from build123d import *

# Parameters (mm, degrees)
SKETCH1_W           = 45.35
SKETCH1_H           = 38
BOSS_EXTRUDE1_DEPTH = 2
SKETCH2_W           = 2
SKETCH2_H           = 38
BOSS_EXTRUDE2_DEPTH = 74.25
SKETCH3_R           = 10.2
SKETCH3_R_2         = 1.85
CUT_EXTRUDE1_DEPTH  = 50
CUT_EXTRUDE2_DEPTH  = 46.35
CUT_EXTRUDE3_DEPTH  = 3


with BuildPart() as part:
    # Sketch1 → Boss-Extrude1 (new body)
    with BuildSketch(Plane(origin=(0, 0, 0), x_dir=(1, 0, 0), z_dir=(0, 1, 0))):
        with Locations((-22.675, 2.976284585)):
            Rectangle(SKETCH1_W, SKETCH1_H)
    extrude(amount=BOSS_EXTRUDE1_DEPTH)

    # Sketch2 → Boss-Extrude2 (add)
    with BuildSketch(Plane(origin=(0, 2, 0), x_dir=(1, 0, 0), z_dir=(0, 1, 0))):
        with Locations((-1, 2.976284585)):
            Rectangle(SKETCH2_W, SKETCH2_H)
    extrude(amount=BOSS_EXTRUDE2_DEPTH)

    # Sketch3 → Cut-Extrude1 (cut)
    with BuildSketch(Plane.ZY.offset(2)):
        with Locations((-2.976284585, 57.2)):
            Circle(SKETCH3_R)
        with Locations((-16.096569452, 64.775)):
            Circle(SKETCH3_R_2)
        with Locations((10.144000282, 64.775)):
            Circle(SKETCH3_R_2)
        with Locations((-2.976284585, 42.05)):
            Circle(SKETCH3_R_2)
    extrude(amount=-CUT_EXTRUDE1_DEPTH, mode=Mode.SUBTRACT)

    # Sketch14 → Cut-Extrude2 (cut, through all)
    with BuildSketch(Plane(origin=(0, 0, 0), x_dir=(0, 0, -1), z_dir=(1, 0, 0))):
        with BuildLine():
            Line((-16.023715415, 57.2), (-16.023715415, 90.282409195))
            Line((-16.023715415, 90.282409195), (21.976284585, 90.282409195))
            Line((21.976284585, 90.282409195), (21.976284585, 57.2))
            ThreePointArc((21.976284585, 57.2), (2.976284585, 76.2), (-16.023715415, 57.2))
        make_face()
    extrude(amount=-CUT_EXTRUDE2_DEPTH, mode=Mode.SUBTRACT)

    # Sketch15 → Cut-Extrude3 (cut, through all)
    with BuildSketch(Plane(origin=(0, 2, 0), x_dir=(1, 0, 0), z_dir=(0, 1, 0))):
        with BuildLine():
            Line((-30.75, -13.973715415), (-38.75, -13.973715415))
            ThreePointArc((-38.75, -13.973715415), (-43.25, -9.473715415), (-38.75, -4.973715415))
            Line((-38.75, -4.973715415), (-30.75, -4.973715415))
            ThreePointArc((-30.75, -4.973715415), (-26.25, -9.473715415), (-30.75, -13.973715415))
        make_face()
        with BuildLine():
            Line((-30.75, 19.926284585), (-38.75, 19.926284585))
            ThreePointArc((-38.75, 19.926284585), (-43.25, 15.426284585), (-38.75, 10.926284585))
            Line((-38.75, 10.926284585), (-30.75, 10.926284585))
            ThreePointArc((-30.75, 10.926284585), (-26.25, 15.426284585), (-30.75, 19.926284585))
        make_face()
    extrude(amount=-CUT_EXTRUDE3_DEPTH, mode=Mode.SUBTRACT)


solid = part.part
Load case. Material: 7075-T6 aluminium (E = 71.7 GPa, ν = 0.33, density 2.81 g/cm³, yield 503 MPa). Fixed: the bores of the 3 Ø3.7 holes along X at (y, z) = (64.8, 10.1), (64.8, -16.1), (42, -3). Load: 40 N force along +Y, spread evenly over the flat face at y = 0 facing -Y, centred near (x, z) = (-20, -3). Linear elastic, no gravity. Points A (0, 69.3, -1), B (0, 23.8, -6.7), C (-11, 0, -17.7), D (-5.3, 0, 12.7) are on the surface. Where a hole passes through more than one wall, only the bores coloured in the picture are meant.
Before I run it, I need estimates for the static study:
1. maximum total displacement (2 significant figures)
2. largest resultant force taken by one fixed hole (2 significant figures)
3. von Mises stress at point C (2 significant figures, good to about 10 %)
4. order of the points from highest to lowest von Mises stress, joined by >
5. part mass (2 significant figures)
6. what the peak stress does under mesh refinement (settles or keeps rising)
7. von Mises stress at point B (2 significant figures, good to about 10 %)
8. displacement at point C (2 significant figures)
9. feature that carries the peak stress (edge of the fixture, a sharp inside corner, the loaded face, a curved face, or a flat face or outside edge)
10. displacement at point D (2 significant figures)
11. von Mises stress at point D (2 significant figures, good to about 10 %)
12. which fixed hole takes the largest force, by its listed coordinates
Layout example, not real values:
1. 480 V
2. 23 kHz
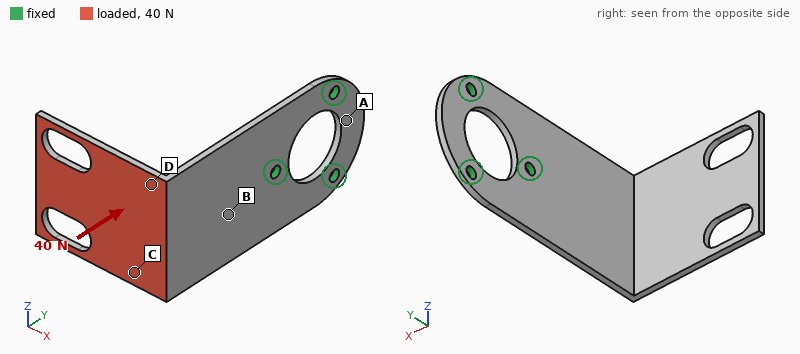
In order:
1. 1.0 mm
2. 32 N
3. 17 MPa
4. B > D > C > A
5. 21 g
6. keeps rising
7. 27 MPa
8. 0.42 mm
9. edge of the fixture
10. 0.39 mm
11. 21 MPa
12. (42, -3)
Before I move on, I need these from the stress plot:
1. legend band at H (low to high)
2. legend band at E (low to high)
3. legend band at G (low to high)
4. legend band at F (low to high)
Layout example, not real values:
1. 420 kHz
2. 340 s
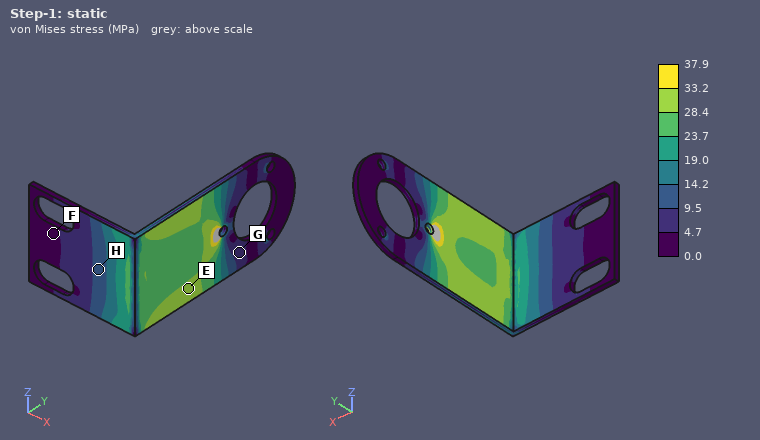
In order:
1. 9.5 to 14.2 MPa
2. 28.4 to 33.2 MPa
3. 4.7 to 9.5 MPa
4. 0.0 to 4.7 MPa
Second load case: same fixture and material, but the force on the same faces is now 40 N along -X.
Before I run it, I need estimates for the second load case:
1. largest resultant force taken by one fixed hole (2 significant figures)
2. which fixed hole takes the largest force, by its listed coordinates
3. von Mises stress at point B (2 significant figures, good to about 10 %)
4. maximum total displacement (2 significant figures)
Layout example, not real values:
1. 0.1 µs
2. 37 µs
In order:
1. 73 N
2. (42, -3)
3. 33 MPa
4. 1.0 mm
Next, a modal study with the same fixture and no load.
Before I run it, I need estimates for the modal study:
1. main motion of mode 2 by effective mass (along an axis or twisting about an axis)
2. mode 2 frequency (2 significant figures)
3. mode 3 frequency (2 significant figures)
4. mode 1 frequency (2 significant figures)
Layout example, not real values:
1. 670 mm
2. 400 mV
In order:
1. along Z
2. 550 Hz
3. 910 Hz
4. 340 Hz
